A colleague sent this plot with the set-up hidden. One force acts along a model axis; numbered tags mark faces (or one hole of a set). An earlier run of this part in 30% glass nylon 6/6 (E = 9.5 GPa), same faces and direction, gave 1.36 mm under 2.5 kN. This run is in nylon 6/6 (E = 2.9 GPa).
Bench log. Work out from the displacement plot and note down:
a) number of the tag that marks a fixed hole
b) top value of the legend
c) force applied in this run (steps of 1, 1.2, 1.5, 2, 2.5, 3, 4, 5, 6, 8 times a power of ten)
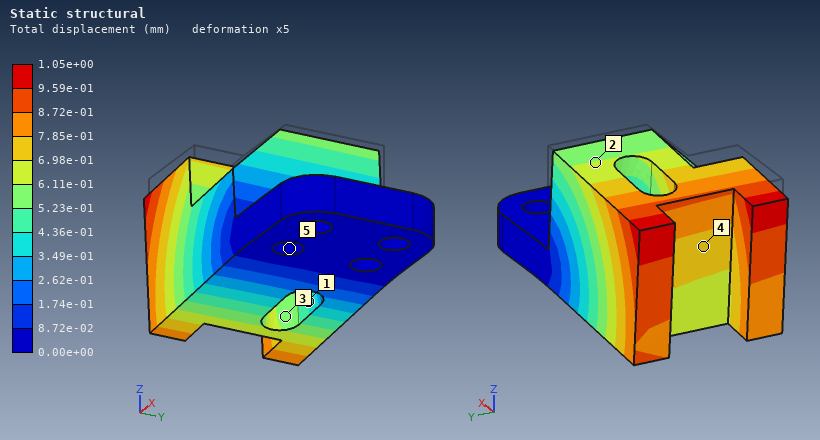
5
1.05e+00 mm
600 N
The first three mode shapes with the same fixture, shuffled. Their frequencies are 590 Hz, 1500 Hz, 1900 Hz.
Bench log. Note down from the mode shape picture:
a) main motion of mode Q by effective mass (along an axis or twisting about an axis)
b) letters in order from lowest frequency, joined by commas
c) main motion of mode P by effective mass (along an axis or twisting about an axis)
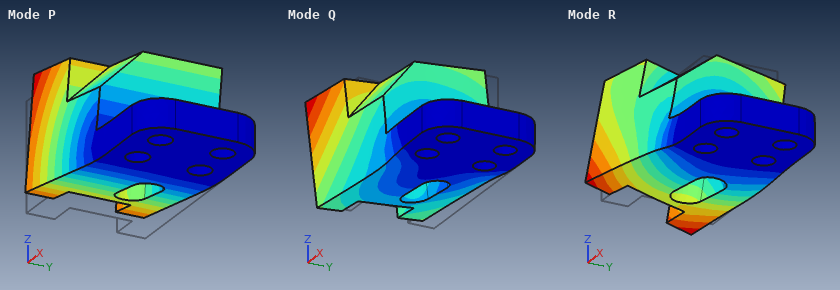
along Y
P, Q, R
along Z
